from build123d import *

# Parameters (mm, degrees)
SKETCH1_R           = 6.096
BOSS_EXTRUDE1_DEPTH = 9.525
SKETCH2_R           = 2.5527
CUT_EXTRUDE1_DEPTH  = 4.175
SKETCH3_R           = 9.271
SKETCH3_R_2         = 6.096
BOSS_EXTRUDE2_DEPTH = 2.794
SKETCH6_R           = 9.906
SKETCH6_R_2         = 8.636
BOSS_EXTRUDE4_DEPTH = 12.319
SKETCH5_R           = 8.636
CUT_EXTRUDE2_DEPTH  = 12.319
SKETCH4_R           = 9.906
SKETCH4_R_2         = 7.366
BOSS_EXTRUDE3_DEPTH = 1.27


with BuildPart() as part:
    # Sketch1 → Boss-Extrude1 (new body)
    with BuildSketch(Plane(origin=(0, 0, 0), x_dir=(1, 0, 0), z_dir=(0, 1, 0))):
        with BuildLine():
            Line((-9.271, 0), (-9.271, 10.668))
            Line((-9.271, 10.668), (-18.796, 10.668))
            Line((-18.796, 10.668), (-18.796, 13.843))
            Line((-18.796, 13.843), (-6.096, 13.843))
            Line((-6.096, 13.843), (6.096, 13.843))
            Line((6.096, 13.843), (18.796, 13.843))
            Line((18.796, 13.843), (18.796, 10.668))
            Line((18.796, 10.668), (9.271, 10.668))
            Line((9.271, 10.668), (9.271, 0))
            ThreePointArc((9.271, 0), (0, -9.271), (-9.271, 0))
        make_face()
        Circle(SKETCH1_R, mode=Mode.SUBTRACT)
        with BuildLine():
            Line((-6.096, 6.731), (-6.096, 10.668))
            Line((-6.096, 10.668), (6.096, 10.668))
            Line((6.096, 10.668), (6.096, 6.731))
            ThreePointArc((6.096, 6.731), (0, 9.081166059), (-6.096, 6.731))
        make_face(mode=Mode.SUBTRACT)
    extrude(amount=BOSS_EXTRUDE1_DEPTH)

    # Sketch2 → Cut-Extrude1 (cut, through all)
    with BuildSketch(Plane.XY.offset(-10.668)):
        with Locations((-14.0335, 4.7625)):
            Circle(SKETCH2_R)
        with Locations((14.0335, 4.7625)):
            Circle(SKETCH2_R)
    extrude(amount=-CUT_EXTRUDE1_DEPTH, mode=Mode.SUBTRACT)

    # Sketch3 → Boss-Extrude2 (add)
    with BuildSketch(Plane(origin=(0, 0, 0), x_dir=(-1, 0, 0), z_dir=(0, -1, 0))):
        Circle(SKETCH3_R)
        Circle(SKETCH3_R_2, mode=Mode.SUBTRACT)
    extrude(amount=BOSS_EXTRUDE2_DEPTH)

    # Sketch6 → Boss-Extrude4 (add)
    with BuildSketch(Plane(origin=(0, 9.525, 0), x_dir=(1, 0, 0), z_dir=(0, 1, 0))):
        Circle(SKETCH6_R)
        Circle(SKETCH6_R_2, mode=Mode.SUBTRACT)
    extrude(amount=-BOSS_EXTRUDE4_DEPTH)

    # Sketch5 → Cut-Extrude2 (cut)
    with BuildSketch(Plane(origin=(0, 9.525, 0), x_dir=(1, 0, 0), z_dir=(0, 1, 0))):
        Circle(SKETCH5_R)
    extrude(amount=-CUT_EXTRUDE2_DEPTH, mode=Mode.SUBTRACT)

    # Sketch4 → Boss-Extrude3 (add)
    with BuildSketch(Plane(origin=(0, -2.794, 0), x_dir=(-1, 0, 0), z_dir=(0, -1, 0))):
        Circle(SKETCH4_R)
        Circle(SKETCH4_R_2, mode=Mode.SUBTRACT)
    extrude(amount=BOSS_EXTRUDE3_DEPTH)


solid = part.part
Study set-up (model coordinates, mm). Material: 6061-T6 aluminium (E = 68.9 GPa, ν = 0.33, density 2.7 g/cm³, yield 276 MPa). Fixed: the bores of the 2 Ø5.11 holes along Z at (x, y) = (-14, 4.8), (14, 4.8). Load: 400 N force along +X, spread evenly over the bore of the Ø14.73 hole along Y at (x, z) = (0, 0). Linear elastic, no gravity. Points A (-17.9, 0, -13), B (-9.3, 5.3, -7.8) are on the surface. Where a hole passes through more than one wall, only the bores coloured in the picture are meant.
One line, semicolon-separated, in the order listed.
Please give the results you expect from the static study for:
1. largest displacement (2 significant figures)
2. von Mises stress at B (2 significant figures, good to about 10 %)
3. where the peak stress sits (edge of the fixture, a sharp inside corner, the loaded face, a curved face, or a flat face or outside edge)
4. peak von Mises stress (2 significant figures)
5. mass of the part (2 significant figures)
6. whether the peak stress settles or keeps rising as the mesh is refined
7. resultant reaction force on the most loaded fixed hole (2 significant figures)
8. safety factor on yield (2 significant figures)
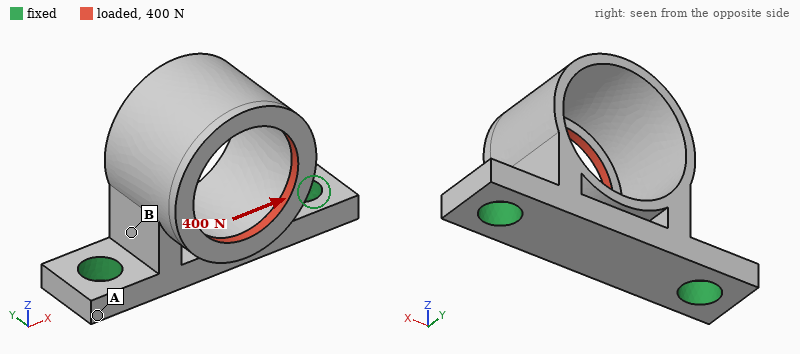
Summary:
98 µm; 45 MPa; the loaded face; 170 MPa; 6.4 g; settles; 320 N; 1.6
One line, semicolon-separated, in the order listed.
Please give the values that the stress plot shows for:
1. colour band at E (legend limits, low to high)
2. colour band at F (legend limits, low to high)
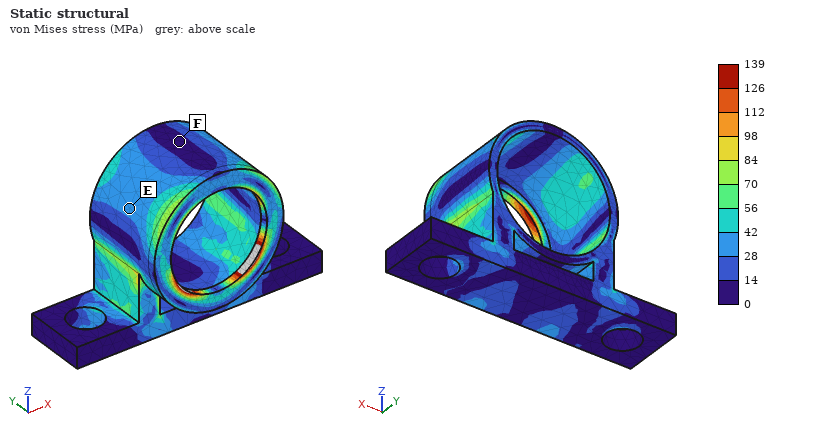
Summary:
28 to 42 MPa; 0 to 14 MPa
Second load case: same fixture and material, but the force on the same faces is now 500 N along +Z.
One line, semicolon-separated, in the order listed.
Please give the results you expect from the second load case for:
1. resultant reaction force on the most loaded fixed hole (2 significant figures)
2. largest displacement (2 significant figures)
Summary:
260 N; 0.11 mm
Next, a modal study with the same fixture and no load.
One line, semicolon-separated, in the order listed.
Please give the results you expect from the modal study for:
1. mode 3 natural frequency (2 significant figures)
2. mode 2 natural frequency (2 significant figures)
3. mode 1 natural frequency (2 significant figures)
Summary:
14 kHz; 6500 Hz; 6400 Hz
